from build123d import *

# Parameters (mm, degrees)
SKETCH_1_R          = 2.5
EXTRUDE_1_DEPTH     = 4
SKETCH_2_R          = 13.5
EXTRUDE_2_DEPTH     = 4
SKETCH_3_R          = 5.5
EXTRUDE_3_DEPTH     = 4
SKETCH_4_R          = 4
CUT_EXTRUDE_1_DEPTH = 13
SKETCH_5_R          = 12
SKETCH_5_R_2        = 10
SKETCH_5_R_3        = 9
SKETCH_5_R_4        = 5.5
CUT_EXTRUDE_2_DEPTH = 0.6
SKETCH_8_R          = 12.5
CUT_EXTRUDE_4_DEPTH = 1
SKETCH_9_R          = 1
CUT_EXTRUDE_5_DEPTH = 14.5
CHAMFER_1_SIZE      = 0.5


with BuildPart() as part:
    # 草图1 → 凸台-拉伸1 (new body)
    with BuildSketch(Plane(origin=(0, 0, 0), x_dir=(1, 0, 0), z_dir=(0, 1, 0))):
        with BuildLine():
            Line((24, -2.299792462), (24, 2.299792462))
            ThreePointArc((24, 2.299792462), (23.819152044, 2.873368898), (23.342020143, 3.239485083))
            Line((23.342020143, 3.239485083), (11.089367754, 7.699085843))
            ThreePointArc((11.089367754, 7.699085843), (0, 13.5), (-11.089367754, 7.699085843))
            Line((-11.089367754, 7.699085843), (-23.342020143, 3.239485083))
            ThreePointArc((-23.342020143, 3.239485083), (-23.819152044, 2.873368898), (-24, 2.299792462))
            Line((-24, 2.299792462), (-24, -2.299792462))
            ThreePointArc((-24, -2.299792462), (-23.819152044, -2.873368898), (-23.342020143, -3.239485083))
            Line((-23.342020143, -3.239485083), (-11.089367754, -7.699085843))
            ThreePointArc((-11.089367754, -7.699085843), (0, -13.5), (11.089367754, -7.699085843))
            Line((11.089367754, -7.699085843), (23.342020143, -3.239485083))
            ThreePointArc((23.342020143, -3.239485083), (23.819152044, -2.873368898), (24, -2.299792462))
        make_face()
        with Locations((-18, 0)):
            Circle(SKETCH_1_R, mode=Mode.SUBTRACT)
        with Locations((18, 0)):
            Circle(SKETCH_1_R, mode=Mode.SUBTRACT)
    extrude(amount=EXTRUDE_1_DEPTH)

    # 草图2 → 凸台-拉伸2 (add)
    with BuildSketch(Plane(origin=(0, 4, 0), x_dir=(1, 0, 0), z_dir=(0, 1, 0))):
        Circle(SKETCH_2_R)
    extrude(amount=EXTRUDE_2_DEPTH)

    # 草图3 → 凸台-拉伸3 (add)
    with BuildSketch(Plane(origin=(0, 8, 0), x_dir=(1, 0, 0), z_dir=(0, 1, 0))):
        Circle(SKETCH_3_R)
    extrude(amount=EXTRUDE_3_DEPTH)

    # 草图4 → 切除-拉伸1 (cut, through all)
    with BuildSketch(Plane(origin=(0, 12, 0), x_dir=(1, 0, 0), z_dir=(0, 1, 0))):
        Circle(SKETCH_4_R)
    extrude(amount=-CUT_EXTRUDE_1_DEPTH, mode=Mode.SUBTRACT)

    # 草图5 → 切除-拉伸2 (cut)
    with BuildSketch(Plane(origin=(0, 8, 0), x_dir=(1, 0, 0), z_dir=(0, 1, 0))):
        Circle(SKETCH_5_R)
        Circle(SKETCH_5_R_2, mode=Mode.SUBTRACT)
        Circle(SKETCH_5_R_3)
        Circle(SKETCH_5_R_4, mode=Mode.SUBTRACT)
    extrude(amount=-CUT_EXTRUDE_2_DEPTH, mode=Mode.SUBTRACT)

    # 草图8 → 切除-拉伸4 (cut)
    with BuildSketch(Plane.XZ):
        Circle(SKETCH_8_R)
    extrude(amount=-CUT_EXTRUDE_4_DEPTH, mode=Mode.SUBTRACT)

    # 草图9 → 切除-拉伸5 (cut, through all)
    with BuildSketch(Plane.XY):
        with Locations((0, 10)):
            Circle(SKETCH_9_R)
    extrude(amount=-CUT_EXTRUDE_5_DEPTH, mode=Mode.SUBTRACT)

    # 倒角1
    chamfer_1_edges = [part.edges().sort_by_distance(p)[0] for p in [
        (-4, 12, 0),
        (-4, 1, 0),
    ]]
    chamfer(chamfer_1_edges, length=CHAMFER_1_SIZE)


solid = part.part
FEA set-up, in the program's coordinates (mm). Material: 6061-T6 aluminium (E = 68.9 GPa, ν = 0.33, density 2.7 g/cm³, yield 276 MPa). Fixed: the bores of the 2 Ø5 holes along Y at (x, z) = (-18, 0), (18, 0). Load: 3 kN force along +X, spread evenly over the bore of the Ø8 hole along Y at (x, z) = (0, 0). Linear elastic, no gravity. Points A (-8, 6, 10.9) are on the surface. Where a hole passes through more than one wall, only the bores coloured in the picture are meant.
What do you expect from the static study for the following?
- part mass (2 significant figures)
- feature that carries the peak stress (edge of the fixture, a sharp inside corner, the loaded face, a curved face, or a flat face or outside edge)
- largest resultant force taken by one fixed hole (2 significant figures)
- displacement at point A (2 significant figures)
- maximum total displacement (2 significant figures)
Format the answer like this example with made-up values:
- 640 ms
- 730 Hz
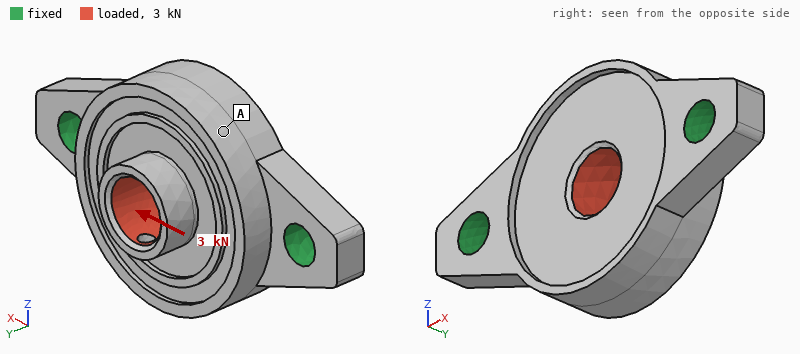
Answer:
- 12 g
- the loaded face
- 1.6 kN
- 4.7 µm
- 15 µm
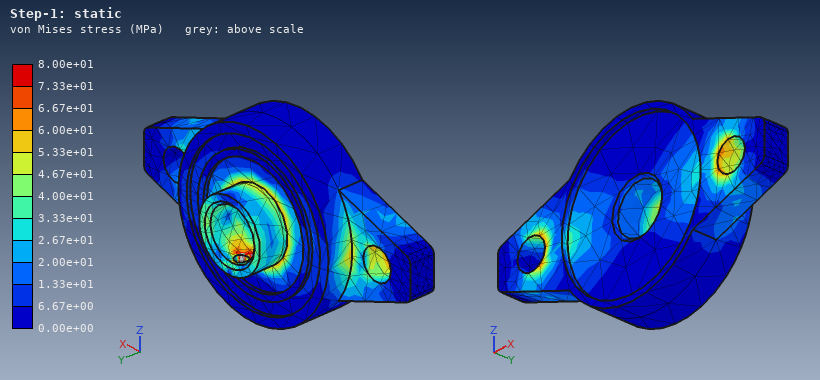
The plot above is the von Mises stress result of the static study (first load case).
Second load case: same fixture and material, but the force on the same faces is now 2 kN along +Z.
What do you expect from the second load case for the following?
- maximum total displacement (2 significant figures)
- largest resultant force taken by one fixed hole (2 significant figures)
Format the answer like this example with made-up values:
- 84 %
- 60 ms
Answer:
- 54 µm
- 1.0 kN
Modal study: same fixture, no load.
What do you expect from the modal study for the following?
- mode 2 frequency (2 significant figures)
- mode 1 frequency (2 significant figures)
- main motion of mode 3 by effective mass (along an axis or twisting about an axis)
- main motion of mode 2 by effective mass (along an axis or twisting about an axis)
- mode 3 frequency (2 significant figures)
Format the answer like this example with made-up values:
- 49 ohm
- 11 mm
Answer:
- 16 kHz
- 10 kHz
- along Z
- along Y
- 28 kHz
